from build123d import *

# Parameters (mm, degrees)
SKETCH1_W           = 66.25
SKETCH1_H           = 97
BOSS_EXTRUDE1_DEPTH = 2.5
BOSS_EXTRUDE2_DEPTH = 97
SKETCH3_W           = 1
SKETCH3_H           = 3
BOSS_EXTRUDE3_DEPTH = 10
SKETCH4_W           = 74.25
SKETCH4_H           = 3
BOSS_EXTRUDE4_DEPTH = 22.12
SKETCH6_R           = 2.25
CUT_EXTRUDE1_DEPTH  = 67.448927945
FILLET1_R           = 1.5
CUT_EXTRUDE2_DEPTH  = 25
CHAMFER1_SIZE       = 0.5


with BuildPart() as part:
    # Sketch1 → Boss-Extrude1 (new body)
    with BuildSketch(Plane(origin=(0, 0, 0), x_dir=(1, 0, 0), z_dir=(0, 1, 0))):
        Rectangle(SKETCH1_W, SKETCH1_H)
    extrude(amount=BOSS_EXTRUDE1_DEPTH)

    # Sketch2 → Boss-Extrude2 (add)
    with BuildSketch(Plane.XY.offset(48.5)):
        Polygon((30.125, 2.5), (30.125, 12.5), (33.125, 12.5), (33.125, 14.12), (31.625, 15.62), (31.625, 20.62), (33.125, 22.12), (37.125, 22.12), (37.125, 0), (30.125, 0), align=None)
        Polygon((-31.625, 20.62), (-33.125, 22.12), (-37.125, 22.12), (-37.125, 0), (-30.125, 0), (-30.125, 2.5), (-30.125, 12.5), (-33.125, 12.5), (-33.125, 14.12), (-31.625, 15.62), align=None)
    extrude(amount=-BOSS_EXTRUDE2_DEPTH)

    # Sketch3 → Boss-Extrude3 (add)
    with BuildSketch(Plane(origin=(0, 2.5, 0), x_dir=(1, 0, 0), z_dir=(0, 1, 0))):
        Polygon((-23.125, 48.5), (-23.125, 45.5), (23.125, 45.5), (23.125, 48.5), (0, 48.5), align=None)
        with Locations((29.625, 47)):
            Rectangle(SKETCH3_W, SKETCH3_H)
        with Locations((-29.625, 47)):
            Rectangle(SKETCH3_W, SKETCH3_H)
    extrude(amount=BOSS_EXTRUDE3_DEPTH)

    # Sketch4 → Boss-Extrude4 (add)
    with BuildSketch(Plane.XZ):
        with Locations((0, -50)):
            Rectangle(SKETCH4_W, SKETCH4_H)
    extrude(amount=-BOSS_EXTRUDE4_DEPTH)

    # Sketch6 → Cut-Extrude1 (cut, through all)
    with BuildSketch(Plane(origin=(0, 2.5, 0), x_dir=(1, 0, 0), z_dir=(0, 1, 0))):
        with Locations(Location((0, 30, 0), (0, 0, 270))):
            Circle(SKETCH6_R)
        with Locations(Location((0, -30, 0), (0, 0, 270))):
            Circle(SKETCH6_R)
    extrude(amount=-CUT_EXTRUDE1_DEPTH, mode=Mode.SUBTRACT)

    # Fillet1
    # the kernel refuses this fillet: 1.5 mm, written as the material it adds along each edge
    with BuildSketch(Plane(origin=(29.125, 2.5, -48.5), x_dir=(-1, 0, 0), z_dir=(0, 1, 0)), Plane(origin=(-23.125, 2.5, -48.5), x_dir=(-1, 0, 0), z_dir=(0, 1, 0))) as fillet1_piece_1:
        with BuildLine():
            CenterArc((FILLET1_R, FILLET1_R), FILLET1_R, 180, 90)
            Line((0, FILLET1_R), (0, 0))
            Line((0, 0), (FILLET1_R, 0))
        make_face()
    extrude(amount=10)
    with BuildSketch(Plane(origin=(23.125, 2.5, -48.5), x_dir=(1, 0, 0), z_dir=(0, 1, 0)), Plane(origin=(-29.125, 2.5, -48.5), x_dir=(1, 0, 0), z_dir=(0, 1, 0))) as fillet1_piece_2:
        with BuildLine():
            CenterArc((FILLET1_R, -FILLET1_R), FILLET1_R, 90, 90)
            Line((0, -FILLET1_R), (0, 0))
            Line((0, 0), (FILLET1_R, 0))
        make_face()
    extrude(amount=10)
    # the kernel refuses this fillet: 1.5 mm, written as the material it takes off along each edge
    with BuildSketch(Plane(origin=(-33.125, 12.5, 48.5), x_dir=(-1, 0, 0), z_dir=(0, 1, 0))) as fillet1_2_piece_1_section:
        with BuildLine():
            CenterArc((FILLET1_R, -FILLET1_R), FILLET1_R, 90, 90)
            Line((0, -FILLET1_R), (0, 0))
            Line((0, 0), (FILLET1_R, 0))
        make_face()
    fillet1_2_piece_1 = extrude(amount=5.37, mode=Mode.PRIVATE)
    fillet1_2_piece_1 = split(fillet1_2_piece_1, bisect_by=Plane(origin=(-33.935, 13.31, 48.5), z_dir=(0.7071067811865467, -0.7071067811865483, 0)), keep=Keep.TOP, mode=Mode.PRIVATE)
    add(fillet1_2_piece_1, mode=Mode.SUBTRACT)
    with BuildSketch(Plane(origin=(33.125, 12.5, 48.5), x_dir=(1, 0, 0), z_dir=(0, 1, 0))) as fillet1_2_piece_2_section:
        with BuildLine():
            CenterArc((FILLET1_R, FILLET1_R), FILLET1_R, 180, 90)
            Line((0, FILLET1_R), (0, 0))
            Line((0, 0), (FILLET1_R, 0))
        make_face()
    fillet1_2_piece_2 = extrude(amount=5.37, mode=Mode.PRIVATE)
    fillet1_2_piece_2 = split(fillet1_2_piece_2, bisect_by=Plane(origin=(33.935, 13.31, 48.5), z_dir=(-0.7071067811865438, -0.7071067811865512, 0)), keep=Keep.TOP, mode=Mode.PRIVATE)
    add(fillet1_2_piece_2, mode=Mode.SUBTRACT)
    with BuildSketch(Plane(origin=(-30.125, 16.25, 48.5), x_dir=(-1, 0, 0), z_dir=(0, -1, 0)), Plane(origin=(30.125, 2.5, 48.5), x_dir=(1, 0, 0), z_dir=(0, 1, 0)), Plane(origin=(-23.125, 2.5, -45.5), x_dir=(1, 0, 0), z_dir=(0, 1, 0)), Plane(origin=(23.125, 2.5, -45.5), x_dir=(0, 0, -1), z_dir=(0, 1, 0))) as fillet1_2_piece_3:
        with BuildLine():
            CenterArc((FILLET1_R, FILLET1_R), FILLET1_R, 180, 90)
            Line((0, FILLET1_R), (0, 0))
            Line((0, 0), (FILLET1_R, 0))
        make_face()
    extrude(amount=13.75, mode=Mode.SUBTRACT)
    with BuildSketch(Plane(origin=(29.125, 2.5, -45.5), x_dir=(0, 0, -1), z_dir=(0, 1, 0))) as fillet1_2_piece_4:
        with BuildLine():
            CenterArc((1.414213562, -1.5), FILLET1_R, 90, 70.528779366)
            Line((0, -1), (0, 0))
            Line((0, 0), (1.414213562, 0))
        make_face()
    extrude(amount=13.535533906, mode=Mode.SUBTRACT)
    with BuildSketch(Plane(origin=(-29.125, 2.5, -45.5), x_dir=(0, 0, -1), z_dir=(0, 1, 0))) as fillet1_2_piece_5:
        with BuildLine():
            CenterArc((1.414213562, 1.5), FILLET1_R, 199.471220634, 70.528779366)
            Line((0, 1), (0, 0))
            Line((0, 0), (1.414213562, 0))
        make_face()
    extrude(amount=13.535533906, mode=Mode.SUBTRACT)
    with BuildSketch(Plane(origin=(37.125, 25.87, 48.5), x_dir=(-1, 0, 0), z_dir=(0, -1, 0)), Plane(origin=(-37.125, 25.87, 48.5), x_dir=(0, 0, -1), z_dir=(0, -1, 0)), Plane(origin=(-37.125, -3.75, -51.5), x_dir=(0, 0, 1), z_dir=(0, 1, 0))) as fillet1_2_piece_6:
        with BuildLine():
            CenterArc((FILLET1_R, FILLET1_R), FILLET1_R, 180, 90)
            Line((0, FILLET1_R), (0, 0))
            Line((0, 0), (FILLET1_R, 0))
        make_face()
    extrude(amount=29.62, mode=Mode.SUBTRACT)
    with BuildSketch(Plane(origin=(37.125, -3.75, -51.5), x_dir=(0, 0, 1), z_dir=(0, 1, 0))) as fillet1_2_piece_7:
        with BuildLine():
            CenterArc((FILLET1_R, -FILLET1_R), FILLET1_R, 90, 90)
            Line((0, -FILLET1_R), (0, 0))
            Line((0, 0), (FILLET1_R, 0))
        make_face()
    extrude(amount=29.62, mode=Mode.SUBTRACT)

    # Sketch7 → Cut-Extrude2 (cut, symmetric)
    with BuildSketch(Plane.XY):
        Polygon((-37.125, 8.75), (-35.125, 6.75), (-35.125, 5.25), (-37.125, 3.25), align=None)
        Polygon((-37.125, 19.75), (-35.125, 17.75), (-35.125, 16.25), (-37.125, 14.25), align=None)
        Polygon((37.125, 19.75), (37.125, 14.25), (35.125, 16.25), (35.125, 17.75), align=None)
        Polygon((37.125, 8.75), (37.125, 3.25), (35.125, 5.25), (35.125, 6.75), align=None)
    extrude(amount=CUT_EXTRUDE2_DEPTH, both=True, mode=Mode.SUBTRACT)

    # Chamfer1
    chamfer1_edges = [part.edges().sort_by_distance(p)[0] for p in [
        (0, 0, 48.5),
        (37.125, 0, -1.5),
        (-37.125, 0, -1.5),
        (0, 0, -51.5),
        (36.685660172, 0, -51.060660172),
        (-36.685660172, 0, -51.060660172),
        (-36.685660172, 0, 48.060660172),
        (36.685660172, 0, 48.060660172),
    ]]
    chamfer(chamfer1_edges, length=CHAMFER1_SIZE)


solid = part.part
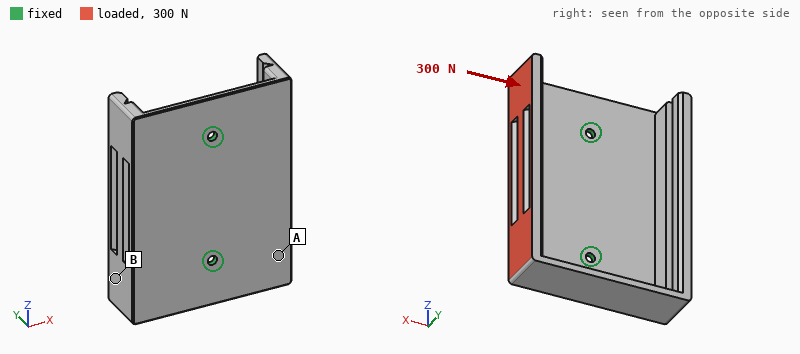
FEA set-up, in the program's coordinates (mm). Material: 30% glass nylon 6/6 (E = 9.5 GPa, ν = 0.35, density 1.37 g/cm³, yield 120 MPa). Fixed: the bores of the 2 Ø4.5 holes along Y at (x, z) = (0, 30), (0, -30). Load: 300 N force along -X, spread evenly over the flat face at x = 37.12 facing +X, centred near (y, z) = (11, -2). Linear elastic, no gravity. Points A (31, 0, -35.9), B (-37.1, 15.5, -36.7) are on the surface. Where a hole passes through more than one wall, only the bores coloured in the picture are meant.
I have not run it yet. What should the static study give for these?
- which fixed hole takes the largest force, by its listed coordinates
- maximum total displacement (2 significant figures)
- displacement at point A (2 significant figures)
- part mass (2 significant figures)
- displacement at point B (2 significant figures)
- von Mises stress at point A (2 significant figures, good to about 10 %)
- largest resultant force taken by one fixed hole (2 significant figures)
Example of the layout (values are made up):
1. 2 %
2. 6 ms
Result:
1. (0, -30)
2. 1.3 mm
3. 0.72 mm
4. 63 g
5. 0.89 mm
6. 7.9 MPa
7. 160 N
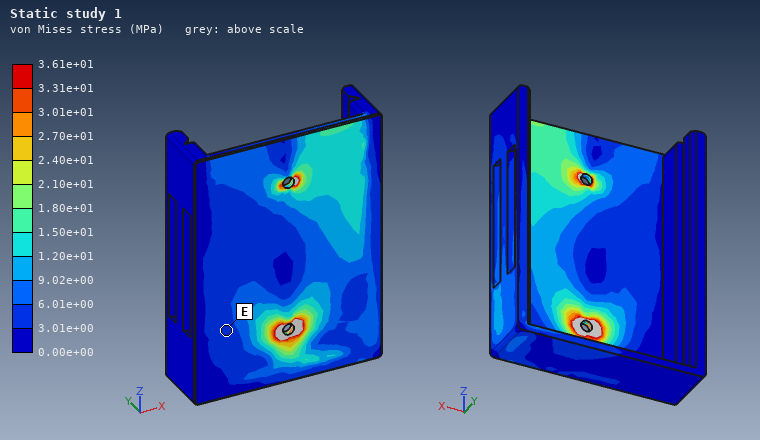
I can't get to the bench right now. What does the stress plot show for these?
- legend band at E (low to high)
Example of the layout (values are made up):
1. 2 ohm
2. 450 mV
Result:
1. 3.01e+00 to 6.01e+00 MPa
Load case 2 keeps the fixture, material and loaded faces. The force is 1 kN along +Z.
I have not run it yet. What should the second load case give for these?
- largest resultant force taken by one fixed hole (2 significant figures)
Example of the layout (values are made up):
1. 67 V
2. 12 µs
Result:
1. 800 N
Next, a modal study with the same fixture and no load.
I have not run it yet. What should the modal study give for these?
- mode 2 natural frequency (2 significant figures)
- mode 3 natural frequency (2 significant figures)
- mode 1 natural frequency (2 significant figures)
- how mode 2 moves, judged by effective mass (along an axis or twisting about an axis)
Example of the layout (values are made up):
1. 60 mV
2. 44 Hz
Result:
1. 540 Hz
2. 680 Hz
3. 280 Hz
4. along Y
